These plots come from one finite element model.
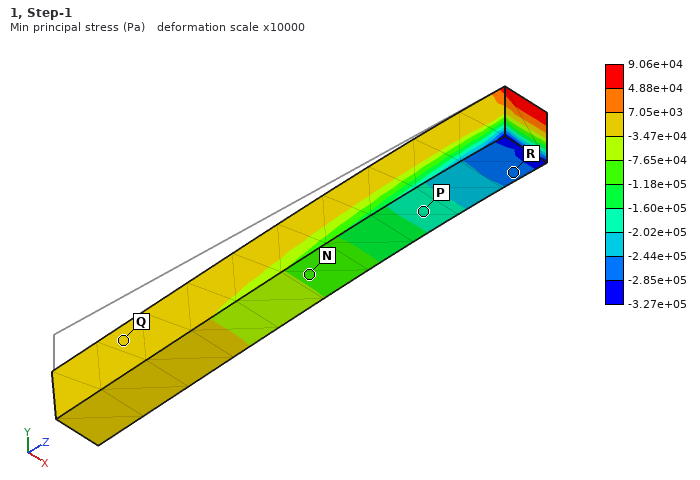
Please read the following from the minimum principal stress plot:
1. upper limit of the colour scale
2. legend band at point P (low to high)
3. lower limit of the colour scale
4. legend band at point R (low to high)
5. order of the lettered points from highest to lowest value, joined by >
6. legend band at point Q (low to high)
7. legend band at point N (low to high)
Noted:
9.06e+04 Pa
-2.02e+05 to -1.60e+05 Pa
-3.27e+05 Pa
-2.85e+05 to -2.44e+05 Pa
Q > N > P > R
-3.47e+04 to 7.05e+03 Pa
-1.18e+05 to -7.65e+04 Pa
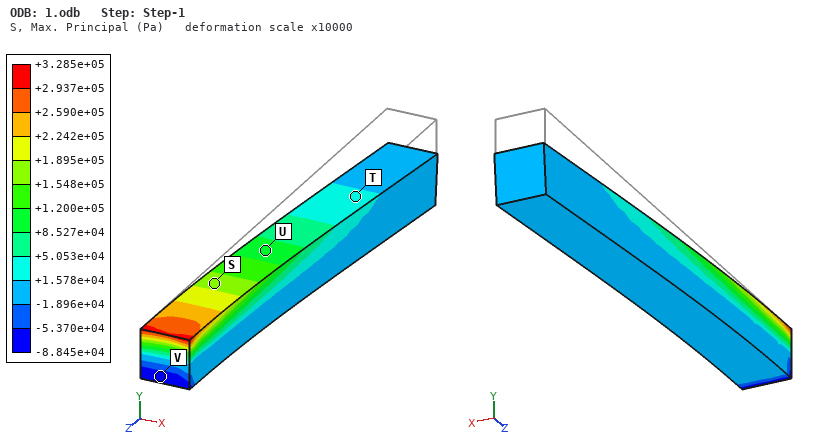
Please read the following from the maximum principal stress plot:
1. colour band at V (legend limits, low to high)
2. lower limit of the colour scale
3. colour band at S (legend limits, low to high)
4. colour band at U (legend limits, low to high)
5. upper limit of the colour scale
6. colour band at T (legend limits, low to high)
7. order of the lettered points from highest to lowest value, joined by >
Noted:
-8.845e+04 to -5.370e+04 Pa
-8.845e+04 Pa
+1.548e+05 to +1.895e+05 Pa
+8.527e+04 to +1.200e+05 Pa
+3.285e+05 Pa
+1.578e+04 to +5.053e+04 Pa
S > U > T > V
